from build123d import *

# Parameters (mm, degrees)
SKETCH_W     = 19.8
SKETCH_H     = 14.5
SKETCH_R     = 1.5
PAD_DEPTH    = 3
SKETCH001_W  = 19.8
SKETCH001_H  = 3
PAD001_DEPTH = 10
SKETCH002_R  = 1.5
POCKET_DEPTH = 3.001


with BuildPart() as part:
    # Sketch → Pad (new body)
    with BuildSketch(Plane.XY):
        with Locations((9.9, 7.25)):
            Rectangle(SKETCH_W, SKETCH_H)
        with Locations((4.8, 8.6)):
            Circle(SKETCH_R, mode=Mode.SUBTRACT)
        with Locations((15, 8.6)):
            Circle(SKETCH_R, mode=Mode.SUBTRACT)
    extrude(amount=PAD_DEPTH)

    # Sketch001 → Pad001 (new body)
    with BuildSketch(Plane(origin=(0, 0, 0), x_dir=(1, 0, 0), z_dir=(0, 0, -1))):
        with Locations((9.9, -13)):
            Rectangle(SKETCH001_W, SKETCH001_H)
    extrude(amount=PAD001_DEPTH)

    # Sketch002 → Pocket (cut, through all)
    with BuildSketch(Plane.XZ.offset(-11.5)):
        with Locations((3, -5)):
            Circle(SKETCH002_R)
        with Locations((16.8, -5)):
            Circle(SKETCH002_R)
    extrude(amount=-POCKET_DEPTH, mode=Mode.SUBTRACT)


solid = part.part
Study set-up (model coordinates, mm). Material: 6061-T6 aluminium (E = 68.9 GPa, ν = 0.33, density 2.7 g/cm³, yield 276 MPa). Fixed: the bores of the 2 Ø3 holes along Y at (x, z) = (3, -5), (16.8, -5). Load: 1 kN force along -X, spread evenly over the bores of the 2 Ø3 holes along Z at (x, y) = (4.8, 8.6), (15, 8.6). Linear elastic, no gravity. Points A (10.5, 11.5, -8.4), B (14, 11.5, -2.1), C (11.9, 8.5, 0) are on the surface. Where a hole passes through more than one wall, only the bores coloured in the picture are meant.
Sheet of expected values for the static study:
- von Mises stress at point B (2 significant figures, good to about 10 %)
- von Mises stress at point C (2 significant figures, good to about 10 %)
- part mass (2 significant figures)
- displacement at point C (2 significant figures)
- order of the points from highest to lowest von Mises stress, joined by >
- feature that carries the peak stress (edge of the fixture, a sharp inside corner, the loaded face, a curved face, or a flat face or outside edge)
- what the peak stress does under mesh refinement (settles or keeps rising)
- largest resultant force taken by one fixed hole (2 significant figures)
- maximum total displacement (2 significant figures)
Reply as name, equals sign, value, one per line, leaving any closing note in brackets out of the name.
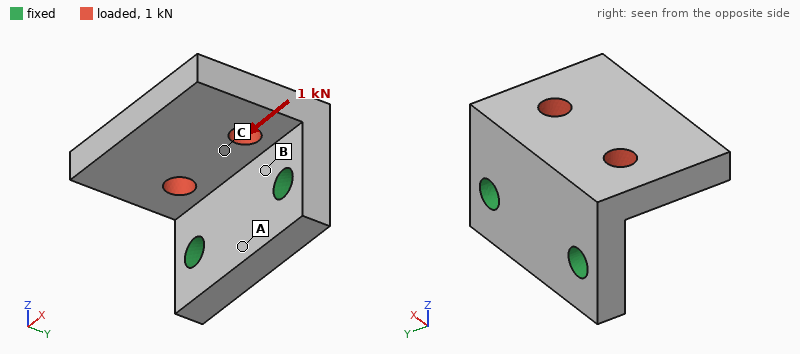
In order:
von Mises stress at point B = 68 MPa
von Mises stress at point C = 46 MPa
part mass = 3.7 g
displacement at point C = 14 µm
order of the points from highest to lowest von Mises stress, joined by > = B > C > A
feature that carries the peak stress = edge of the fixture
what the peak stress does under mesh refinement = keeps rising
largest resultant force taken by one fixed hole = 700 N
maximum total displacement = 32 µm
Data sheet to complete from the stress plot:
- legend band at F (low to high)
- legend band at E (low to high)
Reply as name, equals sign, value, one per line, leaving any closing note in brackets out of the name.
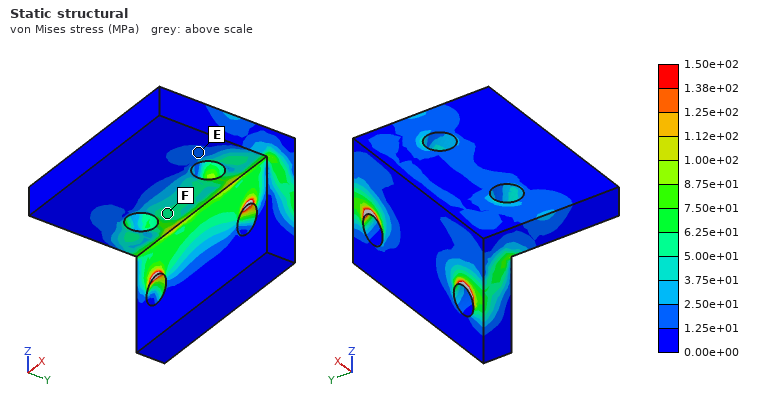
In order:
legend band at F = 5.00e+01 to 6.25e+01 MPa
legend band at E = 1.25e+01 to 2.50e+01 MPa
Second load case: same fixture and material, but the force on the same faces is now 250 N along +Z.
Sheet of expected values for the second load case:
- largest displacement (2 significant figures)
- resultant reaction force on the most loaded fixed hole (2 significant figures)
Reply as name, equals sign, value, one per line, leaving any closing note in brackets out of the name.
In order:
largest displacement = 35 µm
resultant reaction force on the most loaded fixed hole = 130 N
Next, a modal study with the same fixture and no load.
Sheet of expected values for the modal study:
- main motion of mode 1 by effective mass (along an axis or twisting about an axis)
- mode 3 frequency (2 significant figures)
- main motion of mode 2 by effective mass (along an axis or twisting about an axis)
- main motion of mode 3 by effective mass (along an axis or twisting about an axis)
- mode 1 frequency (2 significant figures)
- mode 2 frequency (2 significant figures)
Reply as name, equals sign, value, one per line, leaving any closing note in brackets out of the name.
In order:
main motion of mode 1 by effective mass = along Z
mode 3 frequency = 23 kHz
main motion of mode 2 by effective mass = along X
main motion of mode 3 by effective mass = along X
mode 1 frequency = 8400 Hz
mode 2 frequency = 16 kHz
